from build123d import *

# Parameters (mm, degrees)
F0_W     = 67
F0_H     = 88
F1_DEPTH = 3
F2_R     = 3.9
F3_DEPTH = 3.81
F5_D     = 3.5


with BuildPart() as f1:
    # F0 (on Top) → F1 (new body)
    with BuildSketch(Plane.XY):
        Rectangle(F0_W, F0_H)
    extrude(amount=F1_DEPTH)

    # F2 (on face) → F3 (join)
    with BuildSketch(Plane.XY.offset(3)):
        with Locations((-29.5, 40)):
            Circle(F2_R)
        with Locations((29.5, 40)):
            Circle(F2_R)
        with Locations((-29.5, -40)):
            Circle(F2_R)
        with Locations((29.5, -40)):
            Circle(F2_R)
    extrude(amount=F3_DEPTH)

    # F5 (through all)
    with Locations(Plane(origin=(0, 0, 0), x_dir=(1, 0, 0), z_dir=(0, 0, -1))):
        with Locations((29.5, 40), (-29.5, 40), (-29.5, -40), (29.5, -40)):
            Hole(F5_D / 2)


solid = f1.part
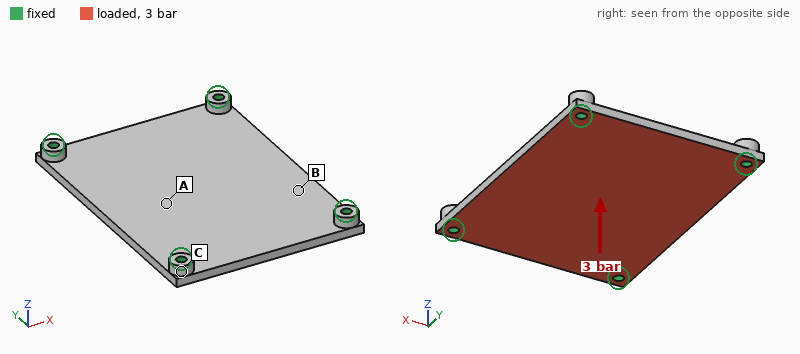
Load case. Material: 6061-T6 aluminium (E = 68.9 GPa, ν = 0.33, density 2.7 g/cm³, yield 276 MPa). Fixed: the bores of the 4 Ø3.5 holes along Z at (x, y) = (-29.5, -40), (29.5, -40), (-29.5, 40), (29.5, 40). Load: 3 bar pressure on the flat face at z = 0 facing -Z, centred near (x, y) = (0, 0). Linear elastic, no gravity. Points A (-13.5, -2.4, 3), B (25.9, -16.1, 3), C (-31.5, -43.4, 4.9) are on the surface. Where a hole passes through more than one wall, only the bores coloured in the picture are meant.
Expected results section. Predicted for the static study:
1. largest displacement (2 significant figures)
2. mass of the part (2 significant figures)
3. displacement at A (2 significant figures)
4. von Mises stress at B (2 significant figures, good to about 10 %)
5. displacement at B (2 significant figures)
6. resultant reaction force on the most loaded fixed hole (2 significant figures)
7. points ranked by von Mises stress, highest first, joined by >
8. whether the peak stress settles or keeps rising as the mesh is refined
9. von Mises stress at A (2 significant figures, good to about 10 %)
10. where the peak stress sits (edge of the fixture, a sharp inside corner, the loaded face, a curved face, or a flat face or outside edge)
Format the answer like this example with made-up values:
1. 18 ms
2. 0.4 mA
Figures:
1. 0.32 mm
2. 49 g
3. 0.31 mm
4. 39 MPa
5. 0.20 mm
6. 460 N
7. A > B > C
8. keeps rising
9. 56 MPa
10. edge of the fixture
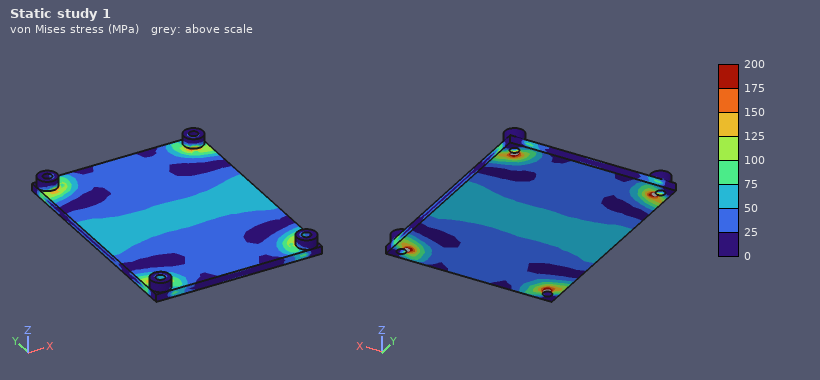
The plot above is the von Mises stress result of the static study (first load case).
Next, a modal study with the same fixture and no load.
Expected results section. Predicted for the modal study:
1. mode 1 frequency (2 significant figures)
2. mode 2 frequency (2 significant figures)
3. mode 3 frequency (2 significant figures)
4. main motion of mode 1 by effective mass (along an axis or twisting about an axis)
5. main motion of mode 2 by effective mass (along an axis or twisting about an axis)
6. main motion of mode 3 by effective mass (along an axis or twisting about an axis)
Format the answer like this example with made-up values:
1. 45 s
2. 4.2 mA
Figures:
1. 2000 Hz
2. 3200 Hz
3. 4500 Hz
4. along Z
5. twisting about Y
6. twisting about X
